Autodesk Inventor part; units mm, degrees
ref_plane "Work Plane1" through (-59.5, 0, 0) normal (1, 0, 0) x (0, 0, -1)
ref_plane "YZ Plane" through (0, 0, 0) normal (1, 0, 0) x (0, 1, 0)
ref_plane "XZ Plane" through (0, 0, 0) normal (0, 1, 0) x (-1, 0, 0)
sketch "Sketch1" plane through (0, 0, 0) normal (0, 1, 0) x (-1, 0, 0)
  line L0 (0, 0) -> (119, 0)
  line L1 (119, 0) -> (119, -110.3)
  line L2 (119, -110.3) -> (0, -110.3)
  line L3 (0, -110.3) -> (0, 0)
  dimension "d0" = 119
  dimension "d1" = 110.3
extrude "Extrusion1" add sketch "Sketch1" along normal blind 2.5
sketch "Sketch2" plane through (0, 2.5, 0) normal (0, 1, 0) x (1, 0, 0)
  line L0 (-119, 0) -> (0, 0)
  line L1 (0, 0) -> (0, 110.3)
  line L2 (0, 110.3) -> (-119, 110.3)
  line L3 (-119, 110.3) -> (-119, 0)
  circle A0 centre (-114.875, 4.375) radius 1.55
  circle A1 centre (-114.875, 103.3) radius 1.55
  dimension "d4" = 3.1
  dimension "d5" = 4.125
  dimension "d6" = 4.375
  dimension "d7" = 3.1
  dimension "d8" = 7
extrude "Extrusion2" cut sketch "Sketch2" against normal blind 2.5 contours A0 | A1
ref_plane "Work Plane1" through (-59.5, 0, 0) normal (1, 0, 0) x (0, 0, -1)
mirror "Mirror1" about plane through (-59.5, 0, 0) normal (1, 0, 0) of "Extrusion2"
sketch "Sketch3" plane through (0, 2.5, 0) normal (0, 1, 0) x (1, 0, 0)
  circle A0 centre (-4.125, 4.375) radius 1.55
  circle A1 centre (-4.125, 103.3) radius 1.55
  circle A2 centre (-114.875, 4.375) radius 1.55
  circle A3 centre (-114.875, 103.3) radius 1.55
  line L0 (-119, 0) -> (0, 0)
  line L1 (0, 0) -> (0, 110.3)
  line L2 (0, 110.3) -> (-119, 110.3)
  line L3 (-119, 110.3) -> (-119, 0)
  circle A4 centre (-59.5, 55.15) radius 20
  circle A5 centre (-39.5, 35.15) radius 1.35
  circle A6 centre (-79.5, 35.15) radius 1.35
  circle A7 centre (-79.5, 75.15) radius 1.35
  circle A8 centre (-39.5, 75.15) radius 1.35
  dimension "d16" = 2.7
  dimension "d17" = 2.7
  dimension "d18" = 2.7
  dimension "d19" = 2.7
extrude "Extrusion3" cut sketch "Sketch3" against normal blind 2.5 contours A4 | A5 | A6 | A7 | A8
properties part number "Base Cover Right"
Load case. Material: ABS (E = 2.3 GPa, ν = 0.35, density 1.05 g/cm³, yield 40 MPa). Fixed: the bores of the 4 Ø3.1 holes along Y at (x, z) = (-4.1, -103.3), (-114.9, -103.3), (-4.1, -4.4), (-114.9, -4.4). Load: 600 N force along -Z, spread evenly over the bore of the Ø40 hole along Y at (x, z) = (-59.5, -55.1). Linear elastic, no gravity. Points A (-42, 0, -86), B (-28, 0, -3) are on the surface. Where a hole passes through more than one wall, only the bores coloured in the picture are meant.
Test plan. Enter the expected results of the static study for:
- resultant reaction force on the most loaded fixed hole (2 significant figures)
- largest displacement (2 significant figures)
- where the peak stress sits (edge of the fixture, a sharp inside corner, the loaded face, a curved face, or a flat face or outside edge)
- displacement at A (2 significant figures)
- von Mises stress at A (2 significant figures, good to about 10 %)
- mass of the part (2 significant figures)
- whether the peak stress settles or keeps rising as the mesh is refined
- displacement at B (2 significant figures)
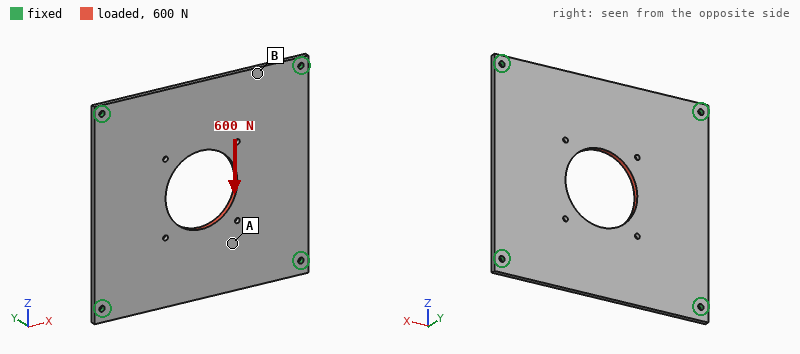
170 N
0.12 mm
edge of the fixture
0.094 mm
1.9 MPa
31 g
keeps rising
0.070 mm
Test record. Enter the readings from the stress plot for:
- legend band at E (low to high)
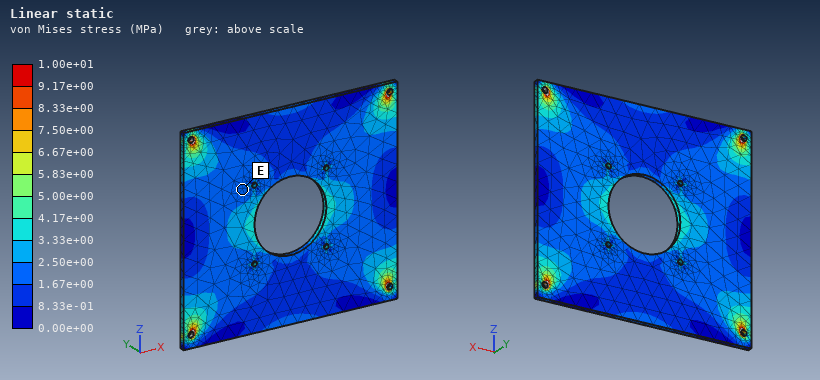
1.67e+00 to 2.50e+00 MPa
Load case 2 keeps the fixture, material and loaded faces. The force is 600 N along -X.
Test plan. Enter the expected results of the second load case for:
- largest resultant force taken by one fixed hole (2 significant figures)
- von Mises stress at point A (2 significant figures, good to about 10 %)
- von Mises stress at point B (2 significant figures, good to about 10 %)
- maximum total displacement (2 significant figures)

170 N
1.9 MPa
2.1 MPa
97 µm
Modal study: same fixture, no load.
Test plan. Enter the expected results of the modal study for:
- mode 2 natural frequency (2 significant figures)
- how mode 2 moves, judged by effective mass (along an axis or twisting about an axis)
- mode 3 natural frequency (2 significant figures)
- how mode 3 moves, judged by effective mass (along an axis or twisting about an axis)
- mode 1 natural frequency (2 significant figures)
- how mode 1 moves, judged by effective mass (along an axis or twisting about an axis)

340 Hz
twisting about X
380 Hz
twisting about Z
210 Hz
along Y
